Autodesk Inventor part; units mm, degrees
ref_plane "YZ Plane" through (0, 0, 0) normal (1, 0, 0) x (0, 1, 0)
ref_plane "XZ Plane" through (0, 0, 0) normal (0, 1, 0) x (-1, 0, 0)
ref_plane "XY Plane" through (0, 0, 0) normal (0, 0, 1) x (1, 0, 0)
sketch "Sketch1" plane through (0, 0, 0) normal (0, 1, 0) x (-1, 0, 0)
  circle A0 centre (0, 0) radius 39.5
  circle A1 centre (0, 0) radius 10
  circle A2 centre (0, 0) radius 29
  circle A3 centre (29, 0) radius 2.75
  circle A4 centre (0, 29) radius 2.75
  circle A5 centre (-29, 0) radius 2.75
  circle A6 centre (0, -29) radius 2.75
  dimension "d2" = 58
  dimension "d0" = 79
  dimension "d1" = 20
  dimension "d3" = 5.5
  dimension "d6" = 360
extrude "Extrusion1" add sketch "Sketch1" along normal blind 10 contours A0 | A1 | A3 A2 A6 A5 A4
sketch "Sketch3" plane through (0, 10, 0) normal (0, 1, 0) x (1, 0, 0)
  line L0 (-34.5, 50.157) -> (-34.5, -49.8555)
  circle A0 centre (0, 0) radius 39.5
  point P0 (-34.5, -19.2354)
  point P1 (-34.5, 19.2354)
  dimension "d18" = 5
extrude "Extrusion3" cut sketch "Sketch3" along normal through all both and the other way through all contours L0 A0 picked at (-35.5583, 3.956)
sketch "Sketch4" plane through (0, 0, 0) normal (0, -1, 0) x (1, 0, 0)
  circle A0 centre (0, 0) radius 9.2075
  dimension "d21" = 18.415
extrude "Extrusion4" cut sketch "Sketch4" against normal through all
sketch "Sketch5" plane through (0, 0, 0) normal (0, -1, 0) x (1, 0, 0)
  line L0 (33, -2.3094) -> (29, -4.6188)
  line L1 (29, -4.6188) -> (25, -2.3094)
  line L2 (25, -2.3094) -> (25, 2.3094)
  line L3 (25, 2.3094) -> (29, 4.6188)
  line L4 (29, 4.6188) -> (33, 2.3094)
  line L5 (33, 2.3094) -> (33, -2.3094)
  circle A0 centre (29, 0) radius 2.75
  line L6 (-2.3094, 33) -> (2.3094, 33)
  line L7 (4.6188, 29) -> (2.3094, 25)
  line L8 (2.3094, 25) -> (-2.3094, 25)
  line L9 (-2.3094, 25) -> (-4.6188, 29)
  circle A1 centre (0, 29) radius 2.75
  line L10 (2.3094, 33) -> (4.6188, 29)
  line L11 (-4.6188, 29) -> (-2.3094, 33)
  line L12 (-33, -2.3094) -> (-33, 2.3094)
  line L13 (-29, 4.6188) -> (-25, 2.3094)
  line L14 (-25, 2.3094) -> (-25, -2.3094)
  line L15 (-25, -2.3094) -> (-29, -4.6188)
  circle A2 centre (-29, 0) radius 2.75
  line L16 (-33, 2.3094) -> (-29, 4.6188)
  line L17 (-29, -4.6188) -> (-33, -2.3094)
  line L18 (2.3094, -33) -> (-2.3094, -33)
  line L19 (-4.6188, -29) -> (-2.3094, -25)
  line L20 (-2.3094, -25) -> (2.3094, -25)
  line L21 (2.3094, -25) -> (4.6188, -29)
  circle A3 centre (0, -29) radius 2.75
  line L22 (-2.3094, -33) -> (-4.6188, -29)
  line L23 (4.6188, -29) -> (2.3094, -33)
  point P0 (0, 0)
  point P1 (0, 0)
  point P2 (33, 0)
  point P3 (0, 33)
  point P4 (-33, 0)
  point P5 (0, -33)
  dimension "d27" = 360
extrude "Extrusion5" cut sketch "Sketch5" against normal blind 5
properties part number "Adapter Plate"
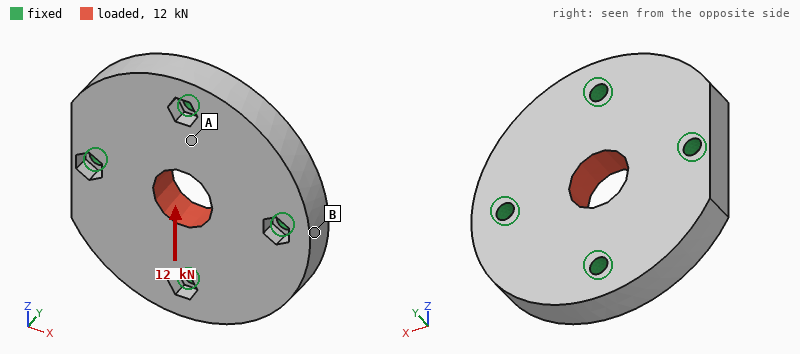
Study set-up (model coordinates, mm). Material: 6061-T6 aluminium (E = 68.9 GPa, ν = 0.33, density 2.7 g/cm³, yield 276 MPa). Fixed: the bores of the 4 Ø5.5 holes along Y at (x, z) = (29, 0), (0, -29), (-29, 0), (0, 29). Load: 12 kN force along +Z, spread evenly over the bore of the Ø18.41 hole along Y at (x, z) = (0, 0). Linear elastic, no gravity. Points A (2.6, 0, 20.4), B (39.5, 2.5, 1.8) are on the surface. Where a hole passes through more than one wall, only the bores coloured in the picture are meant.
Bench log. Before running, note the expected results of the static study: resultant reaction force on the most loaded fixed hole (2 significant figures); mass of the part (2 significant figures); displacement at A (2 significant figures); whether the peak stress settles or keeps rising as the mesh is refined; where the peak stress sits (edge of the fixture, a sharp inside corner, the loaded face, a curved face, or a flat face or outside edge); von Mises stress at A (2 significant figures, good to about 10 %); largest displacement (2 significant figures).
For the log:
3.7 kN
120 g
6.0 µm
keeps rising
edge of the fixture
19 MPa
9.5 µm
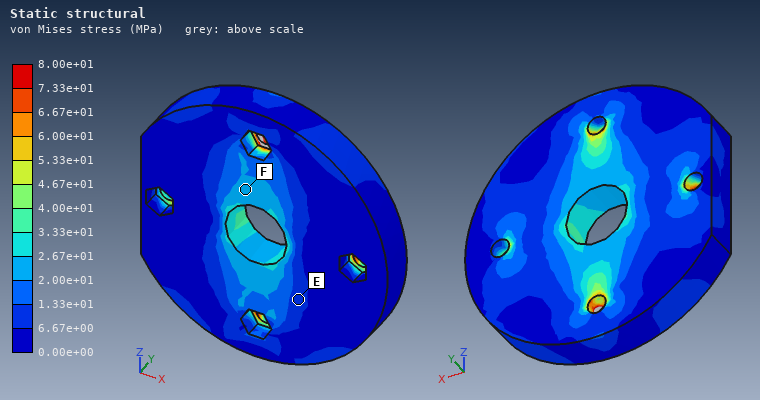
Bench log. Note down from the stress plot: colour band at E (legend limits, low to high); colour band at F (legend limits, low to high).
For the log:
6.67e+00 to 1.33e+01 MPa
2.00e+01 to 2.67e+01 MPa
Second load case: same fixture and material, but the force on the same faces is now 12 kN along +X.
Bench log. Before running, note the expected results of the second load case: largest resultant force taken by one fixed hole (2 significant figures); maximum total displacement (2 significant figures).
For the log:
3.7 kN
9.6 µm
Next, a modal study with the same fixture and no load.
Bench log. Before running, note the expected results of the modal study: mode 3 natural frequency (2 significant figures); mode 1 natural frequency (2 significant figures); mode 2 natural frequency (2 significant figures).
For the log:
13 kHz
11 kHz
13 kHz
